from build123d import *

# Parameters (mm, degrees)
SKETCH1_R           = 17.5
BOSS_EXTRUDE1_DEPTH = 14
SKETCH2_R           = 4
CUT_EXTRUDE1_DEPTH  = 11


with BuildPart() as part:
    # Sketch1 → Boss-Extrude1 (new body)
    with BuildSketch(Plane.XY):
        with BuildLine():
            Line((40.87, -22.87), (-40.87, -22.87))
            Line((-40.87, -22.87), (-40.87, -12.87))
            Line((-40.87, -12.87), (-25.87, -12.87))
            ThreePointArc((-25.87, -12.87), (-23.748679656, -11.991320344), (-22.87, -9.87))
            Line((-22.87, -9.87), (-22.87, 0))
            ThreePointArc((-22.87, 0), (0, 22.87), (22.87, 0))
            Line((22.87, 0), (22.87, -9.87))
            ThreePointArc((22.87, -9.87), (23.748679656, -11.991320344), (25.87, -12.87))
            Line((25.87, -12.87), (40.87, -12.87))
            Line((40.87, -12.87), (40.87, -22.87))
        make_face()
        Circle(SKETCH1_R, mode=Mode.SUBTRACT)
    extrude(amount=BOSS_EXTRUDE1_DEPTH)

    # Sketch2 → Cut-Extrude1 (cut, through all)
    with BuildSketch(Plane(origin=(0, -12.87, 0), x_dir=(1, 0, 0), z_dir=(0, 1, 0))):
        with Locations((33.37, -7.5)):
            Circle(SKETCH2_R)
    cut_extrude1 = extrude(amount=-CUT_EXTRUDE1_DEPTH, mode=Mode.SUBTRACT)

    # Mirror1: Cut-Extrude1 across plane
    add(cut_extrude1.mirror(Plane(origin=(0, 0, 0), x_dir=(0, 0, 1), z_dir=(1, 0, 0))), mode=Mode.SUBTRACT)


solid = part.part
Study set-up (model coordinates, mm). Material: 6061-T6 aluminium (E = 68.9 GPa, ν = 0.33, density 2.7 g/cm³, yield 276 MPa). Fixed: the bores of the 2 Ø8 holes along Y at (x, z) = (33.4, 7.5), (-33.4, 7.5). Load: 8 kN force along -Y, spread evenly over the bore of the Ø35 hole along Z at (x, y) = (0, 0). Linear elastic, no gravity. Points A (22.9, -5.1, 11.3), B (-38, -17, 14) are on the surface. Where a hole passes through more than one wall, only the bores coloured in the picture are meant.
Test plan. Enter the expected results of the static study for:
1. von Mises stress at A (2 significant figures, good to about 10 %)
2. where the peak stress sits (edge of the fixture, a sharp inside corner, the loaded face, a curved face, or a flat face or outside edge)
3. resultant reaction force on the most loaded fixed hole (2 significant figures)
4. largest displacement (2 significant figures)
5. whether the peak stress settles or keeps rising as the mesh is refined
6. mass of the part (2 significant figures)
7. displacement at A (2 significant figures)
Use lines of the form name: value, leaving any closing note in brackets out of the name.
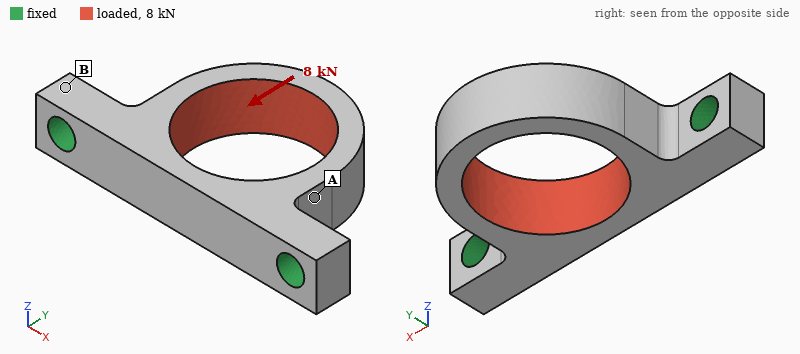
von Mises stress at A: 89 MPa
where the peak stress sits: edge of the fixture
resultant reaction force on the most loaded fixed hole: 4.0 kN
largest displacement: 67 µm
whether the peak stress settles or keeps rising as the mesh is refined: keeps rising
mass of the part: 45 g
displacement at A: 37 µm
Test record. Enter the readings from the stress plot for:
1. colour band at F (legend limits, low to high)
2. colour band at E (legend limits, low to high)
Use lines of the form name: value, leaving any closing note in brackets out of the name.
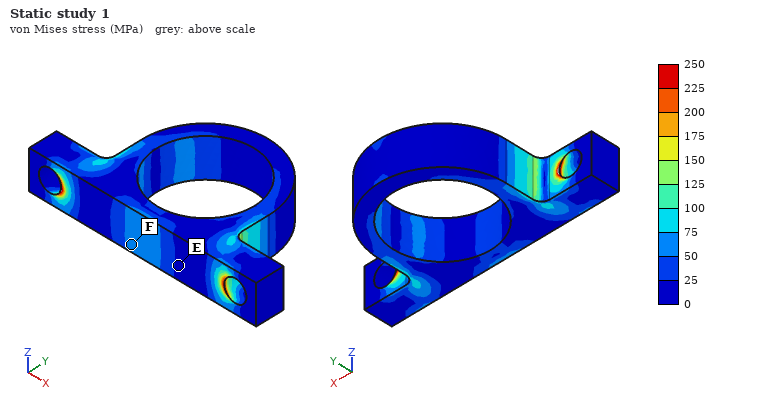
colour band at F: 50 to 75 MPa
colour band at E: 0 to 25 MPa
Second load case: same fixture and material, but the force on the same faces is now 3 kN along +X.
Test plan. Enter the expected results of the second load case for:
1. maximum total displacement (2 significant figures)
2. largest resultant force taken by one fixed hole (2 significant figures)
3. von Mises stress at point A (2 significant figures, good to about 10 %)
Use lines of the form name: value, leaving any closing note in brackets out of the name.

maximum total displacement: 98 µm
largest resultant force taken by one fixed hole: 1.7 kN
von Mises stress at point A: 67 MPa
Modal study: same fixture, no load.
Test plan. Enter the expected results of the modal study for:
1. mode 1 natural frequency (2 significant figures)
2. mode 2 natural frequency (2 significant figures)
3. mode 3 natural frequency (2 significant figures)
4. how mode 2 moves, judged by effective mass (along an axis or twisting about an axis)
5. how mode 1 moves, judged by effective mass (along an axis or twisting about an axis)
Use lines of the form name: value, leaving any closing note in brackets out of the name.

mode 1 natural frequency: 3900 Hz
mode 2 natural frequency: 6000 Hz
mode 3 natural frequency: 9000 Hz
how mode 2 moves, judged by effective mass: along X
how mode 1 moves, judged by effective mass: along Z
